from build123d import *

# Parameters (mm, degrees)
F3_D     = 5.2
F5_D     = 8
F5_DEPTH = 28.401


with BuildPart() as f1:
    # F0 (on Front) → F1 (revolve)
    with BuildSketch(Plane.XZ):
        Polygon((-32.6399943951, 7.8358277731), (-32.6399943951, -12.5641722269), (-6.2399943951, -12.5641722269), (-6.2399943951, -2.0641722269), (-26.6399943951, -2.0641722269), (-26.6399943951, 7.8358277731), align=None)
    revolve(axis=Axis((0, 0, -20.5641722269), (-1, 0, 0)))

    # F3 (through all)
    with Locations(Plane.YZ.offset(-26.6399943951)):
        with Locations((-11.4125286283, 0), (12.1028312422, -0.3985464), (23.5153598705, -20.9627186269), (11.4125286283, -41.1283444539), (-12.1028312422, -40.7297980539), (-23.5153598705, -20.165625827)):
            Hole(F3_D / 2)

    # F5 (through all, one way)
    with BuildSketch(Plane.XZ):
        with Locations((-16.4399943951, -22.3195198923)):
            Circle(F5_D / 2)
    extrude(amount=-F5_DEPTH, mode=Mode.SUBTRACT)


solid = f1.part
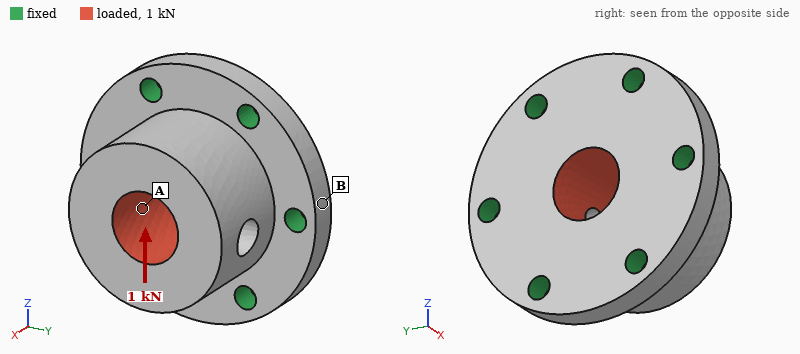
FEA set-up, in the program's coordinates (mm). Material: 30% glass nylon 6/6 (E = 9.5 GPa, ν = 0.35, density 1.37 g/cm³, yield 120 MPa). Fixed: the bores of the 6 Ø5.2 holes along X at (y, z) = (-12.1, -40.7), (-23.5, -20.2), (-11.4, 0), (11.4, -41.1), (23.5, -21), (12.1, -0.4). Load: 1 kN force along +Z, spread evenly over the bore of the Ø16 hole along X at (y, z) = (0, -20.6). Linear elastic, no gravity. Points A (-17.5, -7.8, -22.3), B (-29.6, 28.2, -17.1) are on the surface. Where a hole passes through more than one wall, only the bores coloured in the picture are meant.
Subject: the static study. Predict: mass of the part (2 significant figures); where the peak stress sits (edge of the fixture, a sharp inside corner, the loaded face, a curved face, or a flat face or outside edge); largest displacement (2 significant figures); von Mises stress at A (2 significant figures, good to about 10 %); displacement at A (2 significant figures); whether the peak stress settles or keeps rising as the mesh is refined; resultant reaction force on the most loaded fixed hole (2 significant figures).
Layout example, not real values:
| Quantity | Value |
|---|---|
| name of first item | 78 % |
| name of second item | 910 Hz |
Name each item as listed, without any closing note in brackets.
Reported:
| Quantity | Value |
|---|---|
| mass of the part | 42 g |
| where the peak stress sits | edge of the fixture |
| largest displacement | 14 µm |
| von Mises stress at A | 2.6 MPa |
| displacement at A | 7.9 µm |
| whether the peak stress settles or keeps rising as the mesh is refined | keeps rising |
| resultant reaction force on the most loaded fixed hole | 260 N |
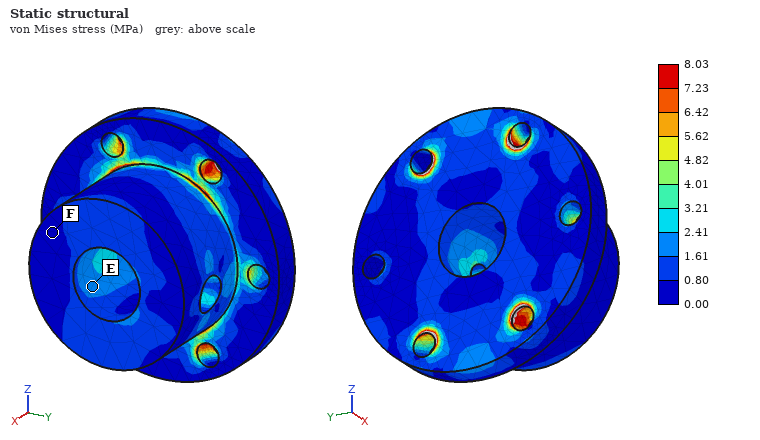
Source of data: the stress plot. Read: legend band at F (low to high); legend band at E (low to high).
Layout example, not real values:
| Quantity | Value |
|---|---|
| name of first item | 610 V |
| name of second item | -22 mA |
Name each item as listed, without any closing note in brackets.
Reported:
| Quantity | Value |
|---|---|
| legend band at F | 0.00 to 0.80 MPa |
| legend band at E | 1.61 to 2.41 MPa |
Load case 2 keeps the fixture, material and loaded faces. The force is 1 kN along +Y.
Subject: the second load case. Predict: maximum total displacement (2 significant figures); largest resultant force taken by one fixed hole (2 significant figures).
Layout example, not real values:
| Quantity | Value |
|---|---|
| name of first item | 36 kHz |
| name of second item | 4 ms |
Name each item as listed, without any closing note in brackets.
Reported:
| Quantity | Value |
|---|---|
| maximum total displacement | 13 µm |
| largest resultant force taken by one fixed hole | 290 N |
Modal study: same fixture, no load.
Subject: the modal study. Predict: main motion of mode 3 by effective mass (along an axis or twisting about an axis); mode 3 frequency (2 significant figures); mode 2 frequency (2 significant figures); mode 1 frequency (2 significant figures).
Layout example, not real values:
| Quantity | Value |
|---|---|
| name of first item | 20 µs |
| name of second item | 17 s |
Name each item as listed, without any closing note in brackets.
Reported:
| Quantity | Value |
|---|---|
| main motion of mode 3 by effective mass | along X |
| mode 3 frequency | 11 kHz |
| mode 2 frequency | 9200 Hz |
| mode 1 frequency | 9100 Hz |
